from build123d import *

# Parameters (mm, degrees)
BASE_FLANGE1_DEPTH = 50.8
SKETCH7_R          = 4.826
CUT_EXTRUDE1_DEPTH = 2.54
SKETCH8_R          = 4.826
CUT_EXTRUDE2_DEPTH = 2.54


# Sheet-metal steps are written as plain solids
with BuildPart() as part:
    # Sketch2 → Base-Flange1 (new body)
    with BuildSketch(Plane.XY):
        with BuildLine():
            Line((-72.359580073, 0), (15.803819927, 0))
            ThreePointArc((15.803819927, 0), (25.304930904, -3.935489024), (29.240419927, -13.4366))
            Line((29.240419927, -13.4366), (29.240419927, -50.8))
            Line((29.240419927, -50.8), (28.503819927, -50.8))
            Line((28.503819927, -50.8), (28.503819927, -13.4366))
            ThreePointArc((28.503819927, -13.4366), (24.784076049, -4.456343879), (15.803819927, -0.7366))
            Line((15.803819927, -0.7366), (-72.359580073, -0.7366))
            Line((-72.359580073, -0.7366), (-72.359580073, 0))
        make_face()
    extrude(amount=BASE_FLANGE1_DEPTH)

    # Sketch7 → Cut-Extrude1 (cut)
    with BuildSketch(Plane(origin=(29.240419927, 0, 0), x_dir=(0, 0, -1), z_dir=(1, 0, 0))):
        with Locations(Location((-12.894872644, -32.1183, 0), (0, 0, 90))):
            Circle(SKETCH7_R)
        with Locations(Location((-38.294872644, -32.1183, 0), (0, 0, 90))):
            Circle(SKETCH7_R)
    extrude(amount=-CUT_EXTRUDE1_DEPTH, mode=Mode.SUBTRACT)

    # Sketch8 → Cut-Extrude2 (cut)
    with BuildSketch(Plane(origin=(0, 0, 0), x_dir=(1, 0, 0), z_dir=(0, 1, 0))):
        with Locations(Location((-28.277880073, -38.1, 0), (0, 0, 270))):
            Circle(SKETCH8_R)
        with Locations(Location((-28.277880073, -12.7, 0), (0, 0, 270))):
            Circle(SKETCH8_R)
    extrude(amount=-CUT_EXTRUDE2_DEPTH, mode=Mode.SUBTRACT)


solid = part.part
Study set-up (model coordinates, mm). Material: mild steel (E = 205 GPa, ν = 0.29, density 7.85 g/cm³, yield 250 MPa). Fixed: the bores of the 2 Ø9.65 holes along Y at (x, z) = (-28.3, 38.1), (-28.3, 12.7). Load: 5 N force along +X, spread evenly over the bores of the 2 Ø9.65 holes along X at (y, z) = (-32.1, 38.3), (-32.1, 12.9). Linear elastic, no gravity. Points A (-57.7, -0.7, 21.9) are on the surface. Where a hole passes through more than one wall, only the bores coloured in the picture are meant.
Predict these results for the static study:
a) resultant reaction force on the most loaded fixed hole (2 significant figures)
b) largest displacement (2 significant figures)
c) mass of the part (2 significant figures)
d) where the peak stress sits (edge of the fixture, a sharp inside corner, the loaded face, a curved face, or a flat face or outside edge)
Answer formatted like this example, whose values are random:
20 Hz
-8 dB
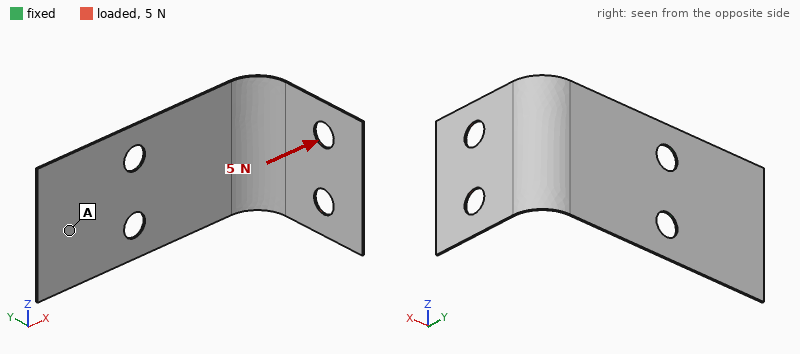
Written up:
2.7 N
1.5 mm
41 g
a flat face or outside edge
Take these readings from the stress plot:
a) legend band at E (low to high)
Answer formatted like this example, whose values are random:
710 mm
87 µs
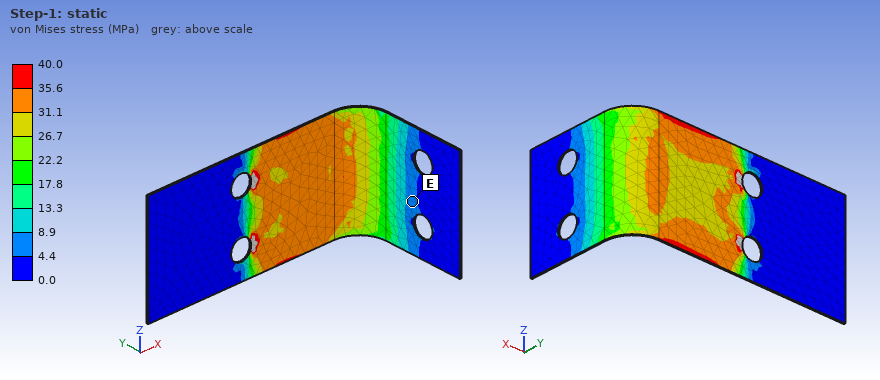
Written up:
4.4 to 8.9 MPa
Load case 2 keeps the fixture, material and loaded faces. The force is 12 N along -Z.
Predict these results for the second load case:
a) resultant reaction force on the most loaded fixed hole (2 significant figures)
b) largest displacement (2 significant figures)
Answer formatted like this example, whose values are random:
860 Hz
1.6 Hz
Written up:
24 N
1.4 mm
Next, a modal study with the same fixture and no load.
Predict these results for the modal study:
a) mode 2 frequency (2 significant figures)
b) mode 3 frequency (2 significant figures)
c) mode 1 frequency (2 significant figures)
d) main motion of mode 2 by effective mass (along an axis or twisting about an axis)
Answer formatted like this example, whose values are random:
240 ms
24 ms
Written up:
160 Hz
250 Hz
83 Hz
along Z
